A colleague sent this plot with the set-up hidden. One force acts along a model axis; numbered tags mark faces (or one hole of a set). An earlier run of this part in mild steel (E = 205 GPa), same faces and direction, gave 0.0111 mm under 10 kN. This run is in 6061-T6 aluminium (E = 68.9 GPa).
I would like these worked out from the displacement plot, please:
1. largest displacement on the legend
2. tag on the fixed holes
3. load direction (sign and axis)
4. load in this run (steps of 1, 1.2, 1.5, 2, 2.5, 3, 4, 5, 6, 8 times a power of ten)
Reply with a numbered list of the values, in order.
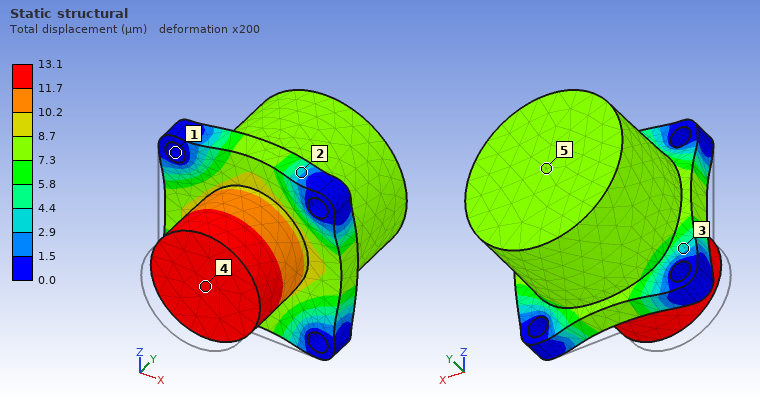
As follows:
1. 13.1 µm
2. 1
3. +Y
4. 4 kN
